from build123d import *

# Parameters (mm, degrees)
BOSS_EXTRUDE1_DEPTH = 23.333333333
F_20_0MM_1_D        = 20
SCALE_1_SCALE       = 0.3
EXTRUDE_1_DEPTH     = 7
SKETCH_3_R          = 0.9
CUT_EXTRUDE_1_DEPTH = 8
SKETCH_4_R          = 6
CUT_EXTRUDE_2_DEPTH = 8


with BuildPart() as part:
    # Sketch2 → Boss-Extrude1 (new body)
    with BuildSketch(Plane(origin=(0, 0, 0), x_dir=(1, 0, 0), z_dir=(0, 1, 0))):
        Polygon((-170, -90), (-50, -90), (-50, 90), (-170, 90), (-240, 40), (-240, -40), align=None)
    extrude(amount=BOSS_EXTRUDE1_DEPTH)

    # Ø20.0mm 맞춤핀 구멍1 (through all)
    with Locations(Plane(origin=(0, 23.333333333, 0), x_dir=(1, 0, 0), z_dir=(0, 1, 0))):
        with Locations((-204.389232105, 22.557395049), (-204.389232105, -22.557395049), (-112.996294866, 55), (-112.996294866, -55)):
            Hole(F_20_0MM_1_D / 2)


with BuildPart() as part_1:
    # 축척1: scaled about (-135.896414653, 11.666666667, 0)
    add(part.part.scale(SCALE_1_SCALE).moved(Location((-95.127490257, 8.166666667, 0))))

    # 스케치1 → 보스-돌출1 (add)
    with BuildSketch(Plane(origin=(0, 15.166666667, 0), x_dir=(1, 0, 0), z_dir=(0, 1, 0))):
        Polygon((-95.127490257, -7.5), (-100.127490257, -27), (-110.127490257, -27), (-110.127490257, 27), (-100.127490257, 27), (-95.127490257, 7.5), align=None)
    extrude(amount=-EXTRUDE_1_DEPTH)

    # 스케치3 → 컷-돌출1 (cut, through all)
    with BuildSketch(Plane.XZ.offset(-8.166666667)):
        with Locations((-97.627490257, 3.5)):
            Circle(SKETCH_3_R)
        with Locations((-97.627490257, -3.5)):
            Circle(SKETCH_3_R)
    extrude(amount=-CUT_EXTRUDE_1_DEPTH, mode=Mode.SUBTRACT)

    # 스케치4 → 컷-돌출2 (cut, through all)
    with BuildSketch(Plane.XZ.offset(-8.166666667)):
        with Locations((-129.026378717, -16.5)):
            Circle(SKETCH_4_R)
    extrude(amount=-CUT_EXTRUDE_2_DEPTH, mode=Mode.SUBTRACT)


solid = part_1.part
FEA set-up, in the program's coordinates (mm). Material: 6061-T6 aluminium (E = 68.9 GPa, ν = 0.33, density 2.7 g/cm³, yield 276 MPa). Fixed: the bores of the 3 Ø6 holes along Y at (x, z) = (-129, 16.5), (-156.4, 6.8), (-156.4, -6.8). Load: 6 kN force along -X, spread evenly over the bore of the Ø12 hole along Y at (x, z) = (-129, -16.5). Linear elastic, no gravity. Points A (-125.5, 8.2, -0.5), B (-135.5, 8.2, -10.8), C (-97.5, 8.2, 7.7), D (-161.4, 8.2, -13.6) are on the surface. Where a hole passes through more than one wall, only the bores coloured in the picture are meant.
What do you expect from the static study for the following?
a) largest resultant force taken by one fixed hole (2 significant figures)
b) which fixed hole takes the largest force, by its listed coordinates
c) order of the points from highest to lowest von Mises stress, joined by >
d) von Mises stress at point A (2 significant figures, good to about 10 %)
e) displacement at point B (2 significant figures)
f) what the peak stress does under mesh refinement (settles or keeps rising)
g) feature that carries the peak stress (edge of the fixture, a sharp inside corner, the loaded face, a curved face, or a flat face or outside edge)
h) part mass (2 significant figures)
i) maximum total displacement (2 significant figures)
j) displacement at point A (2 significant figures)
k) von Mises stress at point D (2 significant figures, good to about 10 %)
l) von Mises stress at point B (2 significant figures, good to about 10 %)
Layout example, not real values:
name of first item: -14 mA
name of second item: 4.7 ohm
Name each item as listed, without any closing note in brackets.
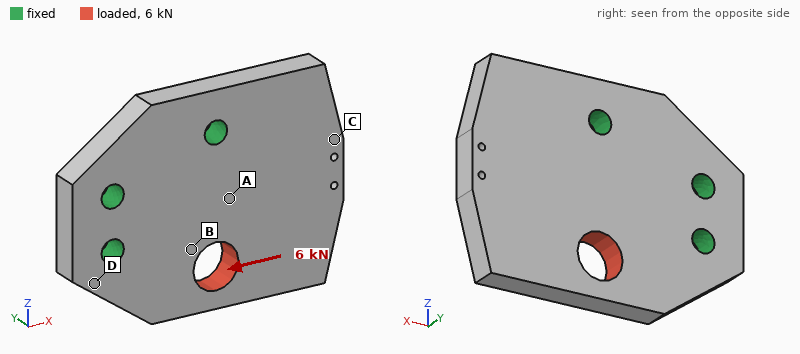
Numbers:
largest resultant force taken by one fixed hole: 5.0 kN
which fixed hole takes the largest force, by its listed coordinates: (-156.4, -6.8)
order of the points from highest to lowest von Mises stress, joined by >: B > D > A > C
von Mises stress at point A: 16 MPa
displacement at point B: 13 µm
what the peak stress does under mesh refinement: keeps rising
feature that carries the peak stress: edge of the fixture
part mass: 62 g
maximum total displacement: 37 µm
displacement at point A: 10.0 µm
von Mises stress at point D: 25 MPa
von Mises stress at point B: 48 MPa
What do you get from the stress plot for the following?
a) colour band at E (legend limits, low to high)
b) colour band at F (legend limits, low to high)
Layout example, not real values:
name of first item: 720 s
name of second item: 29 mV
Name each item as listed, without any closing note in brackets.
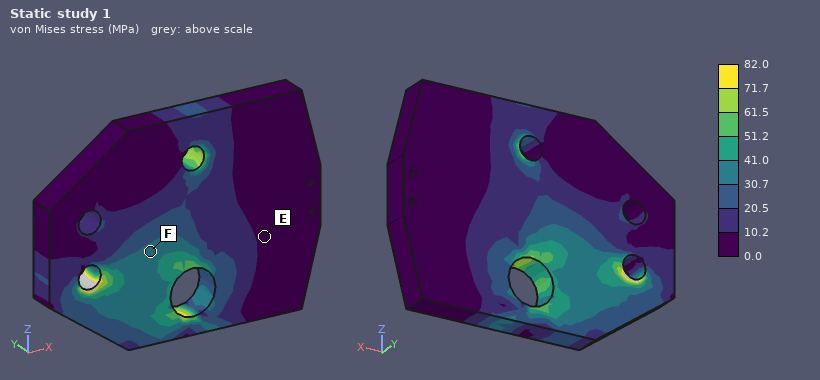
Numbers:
colour band at E: 0.0 to 10.2 MPa
colour band at F: 30.7 to 41.0 MPa
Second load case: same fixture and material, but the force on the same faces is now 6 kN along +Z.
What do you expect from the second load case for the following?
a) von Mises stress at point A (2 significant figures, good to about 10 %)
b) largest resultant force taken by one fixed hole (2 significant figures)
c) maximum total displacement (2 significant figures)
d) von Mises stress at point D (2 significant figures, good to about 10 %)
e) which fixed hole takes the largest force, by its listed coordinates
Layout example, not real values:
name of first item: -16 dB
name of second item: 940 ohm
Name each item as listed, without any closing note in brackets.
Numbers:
von Mises stress at point A: 33 MPa
largest resultant force taken by one fixed hole: 4.8 kN
maximum total displacement: 28 µm
von Mises stress at point D: 10 MPa
which fixed hole takes the largest force, by its listed coordinates: (-129, 16.5)
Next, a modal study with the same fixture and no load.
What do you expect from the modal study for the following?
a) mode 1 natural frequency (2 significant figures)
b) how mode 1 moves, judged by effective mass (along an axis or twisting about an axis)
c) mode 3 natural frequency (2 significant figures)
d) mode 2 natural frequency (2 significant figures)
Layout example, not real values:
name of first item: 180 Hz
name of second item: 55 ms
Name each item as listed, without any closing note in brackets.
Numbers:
mode 1 natural frequency: 3100 Hz
how mode 1 moves, judged by effective mass: along Y
mode 3 natural frequency: 11 kHz
mode 2 natural frequency: 6500 Hz
